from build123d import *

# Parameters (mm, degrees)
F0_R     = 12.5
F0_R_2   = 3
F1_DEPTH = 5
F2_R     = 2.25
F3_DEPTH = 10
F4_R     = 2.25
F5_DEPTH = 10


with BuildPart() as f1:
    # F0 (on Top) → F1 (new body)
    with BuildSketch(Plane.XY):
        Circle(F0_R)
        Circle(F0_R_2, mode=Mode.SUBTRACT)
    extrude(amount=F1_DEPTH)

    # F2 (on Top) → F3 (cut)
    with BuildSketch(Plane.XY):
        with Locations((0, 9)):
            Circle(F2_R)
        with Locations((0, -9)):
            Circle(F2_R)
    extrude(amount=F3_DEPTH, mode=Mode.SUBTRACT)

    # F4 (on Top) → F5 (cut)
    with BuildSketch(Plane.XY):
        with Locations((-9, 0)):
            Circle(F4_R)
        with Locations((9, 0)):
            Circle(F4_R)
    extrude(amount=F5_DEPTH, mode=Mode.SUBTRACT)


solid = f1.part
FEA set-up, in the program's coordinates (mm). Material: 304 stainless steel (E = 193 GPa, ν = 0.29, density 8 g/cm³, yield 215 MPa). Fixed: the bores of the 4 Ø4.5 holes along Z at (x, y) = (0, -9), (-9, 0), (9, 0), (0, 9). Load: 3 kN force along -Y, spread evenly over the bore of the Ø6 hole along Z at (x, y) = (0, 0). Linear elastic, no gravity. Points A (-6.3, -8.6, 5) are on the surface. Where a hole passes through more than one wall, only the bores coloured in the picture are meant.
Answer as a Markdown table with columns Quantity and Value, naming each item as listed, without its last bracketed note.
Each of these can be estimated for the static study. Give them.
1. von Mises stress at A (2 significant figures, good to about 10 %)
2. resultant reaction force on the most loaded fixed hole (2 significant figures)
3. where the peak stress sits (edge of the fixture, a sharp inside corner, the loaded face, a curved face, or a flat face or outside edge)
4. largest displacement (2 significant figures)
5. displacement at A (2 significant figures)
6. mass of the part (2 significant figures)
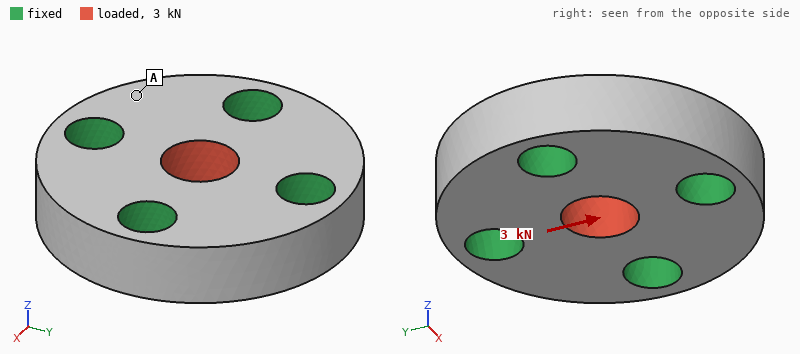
| Quantity | Value |
|---|---|
| von Mises stress at A | 5.4 MPa |
| resultant reaction force on the most loaded fixed hole | 1.0 kN |
| where the peak stress sits | the loaded face |
| largest displacement | 0.95 µm |
| displacement at A | 0.25 µm |
| mass of the part | 16 g |
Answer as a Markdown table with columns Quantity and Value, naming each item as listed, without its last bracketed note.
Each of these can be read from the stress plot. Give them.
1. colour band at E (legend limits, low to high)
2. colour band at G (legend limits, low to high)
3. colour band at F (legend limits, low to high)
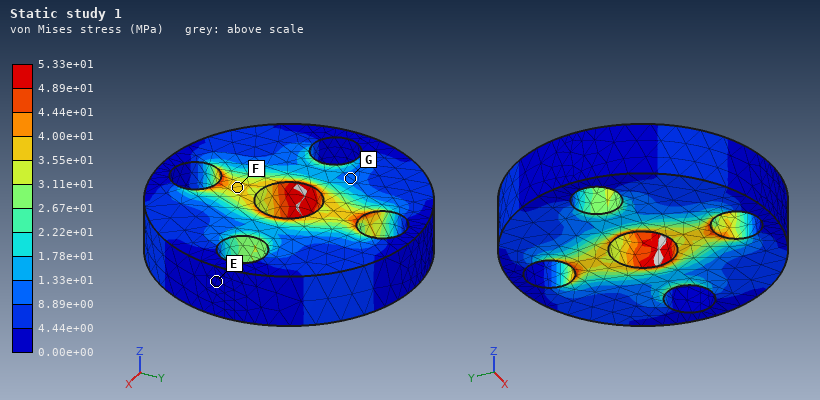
| Quantity | Value |
|---|---|
| colour band at E | 0.00e+00 to 4.44e+00 MPa |
| colour band at G | 8.89e+00 to 1.33e+01 MPa |
| colour band at F | 3.55e+01 to 4.00e+01 MPa |
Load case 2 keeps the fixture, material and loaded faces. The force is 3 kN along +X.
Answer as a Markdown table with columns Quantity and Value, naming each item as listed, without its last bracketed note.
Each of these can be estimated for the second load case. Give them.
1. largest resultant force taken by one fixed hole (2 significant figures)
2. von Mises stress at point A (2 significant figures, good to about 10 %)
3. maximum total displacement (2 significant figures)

| Quantity | Value |
|---|---|
| largest resultant force taken by one fixed hole | 1.0 kN |
| von Mises stress at point A | 5.6 MPa |
| maximum total displacement | 0.95 µm |
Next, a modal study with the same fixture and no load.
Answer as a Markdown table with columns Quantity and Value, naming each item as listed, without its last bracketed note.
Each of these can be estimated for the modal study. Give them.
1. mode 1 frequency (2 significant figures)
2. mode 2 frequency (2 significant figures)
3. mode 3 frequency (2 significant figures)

| Quantity | Value |
|---|---|
| mode 1 frequency | 95 kHz |
| mode 2 frequency | 96 kHz |
| mode 3 frequency | 96 kHz |
